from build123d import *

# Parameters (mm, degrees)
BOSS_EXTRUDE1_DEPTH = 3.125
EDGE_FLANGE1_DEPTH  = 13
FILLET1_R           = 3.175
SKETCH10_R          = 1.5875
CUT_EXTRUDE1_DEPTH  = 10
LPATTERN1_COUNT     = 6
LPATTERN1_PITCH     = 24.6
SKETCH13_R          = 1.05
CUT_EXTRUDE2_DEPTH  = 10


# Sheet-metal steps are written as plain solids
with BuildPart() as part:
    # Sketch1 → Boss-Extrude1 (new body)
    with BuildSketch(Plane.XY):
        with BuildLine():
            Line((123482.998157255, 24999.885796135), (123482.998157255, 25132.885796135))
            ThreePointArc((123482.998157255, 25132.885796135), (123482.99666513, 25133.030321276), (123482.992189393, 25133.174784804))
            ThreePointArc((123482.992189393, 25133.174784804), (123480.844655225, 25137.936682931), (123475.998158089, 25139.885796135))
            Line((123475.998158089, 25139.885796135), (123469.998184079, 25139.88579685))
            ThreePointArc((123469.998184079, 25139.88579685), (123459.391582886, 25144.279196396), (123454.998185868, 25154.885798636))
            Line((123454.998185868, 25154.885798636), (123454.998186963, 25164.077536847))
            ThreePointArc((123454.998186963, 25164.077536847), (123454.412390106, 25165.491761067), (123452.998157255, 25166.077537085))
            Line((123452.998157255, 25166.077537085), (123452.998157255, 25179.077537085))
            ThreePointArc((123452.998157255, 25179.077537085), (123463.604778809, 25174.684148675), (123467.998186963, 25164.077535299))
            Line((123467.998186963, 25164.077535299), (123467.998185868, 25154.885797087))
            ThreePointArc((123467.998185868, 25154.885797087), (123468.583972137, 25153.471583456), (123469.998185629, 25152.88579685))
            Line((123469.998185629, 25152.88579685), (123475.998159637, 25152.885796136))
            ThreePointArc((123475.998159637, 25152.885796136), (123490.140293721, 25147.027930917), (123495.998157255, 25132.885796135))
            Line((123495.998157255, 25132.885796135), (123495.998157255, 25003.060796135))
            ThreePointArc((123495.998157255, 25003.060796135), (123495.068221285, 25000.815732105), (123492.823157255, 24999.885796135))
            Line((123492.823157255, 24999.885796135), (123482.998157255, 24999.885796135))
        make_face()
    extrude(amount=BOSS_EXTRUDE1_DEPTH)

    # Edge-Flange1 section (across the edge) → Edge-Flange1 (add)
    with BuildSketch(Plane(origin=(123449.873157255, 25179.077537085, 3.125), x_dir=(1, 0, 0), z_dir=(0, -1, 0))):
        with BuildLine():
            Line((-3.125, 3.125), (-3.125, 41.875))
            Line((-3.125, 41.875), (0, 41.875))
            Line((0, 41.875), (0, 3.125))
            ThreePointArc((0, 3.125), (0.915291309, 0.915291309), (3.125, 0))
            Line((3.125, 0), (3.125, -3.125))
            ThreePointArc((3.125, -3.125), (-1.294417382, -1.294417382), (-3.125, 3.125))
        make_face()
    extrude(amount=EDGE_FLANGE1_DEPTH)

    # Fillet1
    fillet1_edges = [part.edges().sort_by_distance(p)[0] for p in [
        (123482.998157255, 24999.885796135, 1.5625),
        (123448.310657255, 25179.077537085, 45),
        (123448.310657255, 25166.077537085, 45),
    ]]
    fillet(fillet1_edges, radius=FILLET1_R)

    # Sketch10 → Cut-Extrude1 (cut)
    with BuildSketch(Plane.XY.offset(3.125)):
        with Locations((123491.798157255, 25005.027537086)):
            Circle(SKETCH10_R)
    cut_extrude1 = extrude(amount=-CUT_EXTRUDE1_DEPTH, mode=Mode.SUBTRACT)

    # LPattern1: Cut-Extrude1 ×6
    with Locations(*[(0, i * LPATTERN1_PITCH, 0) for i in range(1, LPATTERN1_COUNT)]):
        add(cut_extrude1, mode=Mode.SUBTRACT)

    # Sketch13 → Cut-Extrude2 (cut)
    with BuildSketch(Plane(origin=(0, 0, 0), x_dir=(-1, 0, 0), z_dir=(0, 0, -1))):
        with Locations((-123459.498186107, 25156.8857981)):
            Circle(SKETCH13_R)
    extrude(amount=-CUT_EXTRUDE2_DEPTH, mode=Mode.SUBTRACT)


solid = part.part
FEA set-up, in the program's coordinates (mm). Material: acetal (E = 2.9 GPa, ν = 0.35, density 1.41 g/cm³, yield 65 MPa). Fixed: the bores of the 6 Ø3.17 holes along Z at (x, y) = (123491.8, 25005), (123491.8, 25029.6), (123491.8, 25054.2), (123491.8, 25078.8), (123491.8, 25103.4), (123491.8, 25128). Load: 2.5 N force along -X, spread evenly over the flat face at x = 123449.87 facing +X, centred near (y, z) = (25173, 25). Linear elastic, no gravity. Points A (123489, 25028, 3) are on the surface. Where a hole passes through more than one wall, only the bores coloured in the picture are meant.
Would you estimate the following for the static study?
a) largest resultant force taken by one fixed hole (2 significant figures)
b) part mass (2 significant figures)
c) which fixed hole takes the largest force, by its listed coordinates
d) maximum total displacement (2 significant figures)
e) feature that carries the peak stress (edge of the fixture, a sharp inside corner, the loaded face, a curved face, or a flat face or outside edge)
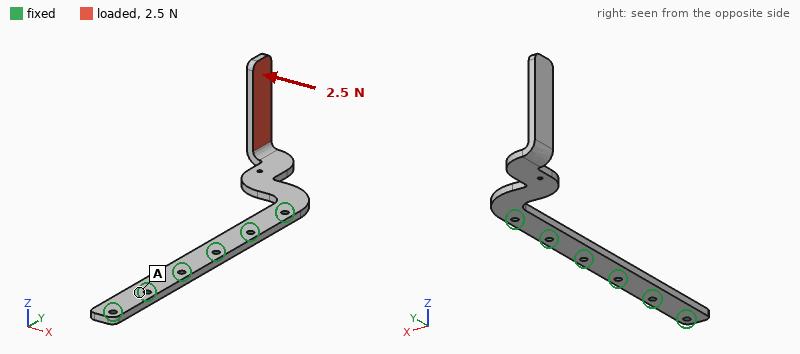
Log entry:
6.8 N
14 g
(123491.8, 25128)
2.2 mm
a curved face
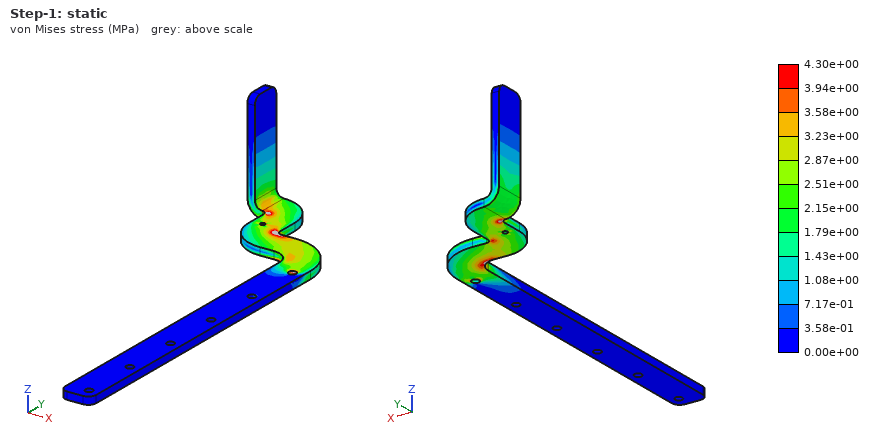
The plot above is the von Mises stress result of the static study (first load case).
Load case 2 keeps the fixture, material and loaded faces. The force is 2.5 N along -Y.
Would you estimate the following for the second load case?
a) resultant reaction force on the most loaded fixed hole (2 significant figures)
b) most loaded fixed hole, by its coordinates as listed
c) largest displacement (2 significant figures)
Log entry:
4.8 N
(123491.8, 25103.4)
2.0 mm
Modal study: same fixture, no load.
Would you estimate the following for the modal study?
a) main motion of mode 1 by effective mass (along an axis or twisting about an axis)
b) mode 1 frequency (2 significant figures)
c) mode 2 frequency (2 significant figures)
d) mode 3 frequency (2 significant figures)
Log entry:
along Z
82 Hz
150 Hz
290 Hz
